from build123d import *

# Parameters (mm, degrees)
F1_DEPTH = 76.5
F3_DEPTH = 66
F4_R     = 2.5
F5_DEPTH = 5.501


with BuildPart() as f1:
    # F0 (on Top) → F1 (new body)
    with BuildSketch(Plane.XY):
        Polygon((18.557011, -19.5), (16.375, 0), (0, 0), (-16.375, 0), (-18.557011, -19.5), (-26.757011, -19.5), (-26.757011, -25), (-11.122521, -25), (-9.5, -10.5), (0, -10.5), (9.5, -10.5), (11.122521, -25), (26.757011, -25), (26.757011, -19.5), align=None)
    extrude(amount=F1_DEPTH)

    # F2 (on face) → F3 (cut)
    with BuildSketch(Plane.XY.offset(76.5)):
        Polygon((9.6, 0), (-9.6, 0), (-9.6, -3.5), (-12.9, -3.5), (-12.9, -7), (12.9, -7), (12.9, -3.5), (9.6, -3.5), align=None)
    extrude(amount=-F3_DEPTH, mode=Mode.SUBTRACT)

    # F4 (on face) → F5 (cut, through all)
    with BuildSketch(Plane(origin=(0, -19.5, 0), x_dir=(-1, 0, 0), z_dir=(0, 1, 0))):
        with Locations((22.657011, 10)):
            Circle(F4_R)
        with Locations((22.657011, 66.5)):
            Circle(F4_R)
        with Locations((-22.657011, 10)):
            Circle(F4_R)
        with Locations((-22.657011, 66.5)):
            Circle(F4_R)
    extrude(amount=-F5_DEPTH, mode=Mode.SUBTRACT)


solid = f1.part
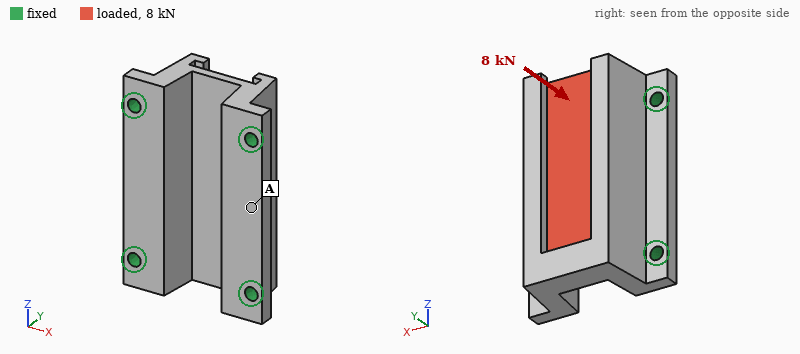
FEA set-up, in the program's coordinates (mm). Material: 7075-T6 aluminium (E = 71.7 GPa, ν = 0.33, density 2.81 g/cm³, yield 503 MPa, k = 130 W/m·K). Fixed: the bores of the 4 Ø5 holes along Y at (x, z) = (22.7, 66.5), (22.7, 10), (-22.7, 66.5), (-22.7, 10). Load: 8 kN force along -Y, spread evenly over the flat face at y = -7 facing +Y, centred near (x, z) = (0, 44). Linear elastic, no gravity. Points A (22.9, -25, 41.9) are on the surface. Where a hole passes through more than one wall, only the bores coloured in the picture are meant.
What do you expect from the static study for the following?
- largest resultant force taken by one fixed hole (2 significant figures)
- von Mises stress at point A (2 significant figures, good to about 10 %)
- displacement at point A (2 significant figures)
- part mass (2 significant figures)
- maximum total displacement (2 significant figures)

3.1 kN
14 MPa
15 µm
110 g
34 µm
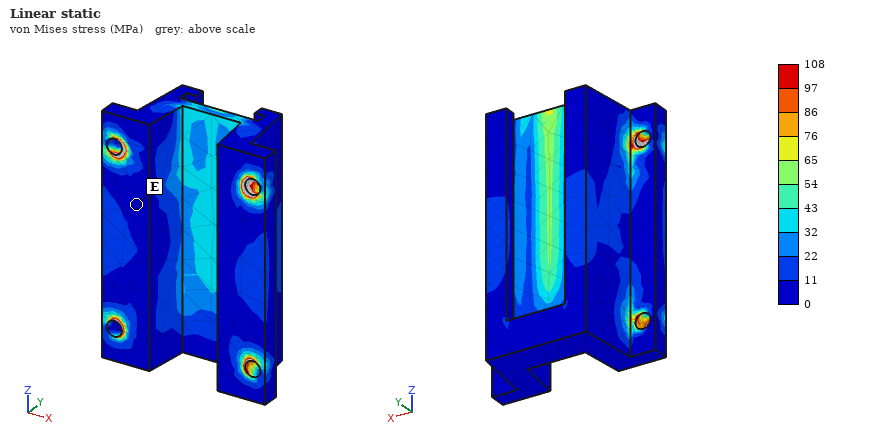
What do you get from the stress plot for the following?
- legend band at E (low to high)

0 to 11 MPa
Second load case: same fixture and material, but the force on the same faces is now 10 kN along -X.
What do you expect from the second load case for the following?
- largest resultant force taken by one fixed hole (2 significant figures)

3.2 kN
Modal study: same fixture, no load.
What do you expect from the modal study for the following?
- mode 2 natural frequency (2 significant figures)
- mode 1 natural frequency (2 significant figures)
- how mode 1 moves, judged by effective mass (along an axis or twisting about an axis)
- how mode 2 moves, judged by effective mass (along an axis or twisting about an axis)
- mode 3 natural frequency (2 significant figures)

12 kHz
8600 Hz
along X
along Y
12 kHz
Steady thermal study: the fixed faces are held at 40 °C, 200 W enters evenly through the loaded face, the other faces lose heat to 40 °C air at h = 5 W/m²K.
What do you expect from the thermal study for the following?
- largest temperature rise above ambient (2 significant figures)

65 K
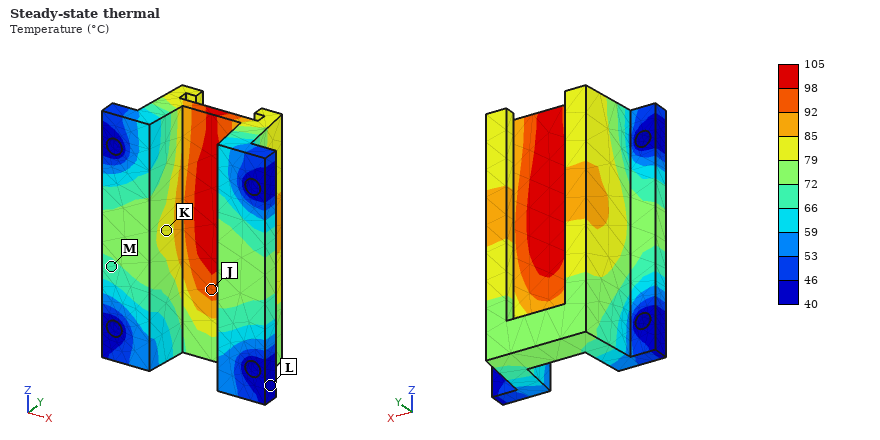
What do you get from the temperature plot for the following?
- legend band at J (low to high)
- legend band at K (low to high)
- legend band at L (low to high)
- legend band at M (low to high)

92 to 98 °C
79 to 85 °C
40 to 46 °C
66 to 72 °C
